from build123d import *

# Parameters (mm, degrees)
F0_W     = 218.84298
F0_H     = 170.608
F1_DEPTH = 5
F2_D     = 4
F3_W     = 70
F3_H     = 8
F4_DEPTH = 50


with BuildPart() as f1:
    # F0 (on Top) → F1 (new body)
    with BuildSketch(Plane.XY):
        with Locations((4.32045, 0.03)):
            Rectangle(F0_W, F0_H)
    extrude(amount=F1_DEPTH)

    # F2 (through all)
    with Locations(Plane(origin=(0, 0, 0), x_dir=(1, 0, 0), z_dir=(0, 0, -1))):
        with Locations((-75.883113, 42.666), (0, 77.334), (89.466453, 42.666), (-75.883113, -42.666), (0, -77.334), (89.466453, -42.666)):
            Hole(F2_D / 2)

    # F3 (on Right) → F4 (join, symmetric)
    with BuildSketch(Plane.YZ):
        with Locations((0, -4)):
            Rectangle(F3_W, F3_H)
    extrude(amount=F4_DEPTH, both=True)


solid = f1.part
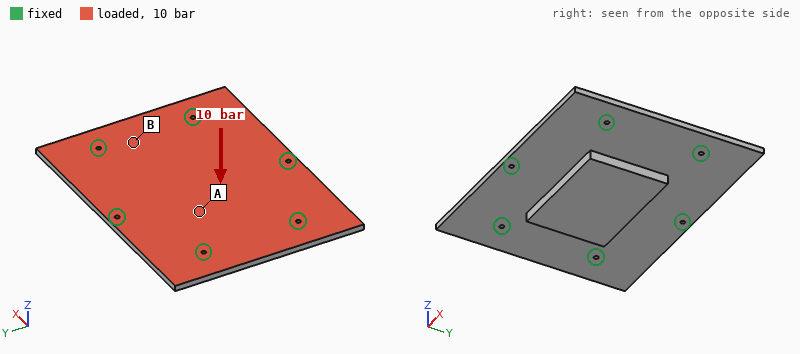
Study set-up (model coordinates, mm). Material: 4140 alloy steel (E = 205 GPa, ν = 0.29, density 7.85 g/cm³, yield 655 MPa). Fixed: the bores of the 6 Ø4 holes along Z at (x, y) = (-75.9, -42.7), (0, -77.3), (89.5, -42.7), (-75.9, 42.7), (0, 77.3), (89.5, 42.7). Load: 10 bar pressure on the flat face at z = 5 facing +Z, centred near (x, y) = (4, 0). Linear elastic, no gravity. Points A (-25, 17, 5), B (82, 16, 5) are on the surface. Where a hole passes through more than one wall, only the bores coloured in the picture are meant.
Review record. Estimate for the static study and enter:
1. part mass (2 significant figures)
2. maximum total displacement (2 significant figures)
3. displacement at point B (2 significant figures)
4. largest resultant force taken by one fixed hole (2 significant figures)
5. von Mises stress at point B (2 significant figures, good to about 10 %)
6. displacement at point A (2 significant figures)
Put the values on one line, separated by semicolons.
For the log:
1.9 kg; 0.22 mm; 0.11 mm; 6.9 kN; 80 MPa; 0.16 mm
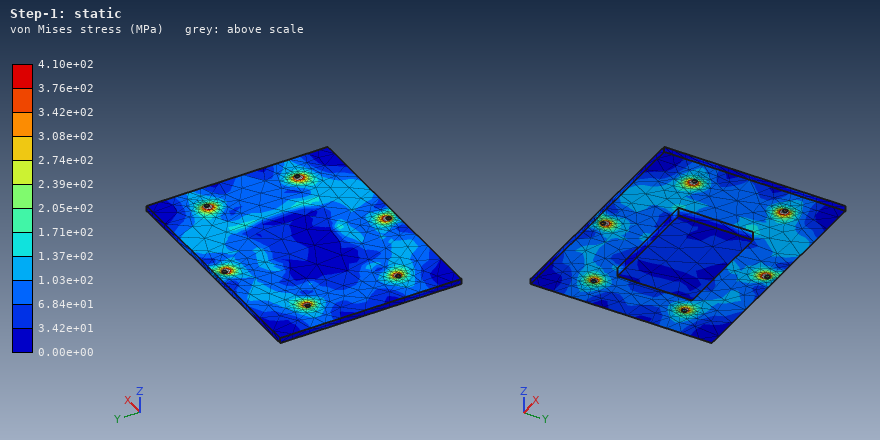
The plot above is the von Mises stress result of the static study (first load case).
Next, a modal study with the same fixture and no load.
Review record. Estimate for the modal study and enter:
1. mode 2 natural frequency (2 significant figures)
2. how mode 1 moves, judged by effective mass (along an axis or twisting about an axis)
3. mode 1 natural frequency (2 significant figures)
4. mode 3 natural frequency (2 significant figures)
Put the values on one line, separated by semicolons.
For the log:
2100 Hz; along Z; 1400 Hz; 2100 Hz
